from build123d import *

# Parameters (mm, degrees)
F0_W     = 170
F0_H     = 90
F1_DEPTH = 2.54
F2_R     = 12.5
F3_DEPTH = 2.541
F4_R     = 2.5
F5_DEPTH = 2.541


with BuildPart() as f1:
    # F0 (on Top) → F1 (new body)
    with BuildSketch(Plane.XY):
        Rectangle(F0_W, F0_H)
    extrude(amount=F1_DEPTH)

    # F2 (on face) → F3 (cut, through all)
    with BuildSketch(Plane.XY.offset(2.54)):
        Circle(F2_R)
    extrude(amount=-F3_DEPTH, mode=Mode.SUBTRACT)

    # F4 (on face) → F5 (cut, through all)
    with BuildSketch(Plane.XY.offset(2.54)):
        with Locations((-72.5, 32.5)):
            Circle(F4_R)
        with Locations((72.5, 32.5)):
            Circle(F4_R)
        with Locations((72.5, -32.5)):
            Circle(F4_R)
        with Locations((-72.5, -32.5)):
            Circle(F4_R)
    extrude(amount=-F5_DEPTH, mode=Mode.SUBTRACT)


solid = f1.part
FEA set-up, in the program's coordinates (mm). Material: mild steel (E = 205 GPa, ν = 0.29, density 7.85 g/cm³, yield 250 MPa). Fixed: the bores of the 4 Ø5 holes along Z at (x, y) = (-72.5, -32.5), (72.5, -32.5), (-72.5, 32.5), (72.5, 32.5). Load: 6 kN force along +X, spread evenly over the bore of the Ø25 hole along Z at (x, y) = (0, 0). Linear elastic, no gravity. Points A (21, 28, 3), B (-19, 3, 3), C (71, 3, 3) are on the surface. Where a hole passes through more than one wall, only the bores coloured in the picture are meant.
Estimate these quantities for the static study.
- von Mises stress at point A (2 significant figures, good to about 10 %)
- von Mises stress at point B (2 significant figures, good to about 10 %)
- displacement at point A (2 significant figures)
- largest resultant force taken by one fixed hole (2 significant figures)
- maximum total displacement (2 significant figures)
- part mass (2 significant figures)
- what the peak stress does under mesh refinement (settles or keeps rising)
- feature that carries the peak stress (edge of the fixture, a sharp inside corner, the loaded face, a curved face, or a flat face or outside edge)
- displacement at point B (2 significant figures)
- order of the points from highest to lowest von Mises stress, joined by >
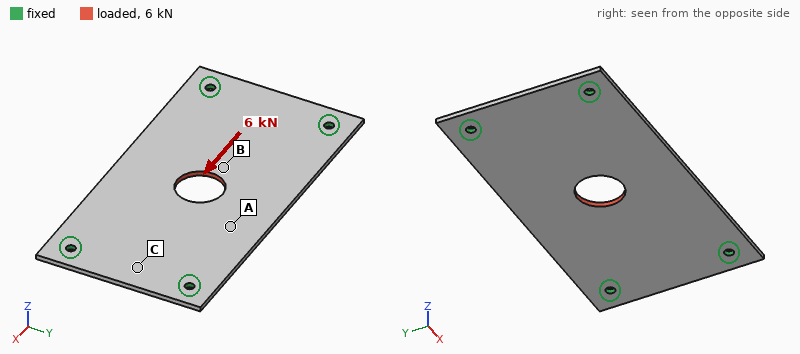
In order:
12 MPa
28 MPa
4.5 µm
1.5 kN
7.9 µm
290 g
keeps rising
edge of the fixture
6.7 µm
B > A > C
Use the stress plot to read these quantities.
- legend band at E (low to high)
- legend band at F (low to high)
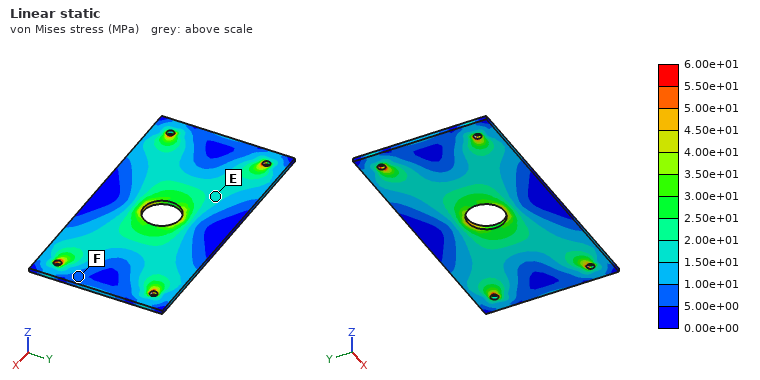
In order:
1.50e+01 to 2.00e+01 MPa
5.00e+00 to 1.00e+01 MPa
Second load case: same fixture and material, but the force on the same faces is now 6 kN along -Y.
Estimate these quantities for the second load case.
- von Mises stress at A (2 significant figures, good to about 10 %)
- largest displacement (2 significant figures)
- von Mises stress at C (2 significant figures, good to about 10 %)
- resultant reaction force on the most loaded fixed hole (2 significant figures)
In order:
23 MPa
19 µm
15 MPa
2.1 kN
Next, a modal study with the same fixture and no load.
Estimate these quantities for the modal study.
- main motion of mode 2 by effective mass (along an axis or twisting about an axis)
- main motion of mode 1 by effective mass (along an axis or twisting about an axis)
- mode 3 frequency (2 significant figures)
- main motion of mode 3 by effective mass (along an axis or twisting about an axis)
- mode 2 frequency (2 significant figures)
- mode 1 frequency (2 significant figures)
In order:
twisting about X
along Z
1600 Hz
twisting about Y
930 Hz
590 Hz
